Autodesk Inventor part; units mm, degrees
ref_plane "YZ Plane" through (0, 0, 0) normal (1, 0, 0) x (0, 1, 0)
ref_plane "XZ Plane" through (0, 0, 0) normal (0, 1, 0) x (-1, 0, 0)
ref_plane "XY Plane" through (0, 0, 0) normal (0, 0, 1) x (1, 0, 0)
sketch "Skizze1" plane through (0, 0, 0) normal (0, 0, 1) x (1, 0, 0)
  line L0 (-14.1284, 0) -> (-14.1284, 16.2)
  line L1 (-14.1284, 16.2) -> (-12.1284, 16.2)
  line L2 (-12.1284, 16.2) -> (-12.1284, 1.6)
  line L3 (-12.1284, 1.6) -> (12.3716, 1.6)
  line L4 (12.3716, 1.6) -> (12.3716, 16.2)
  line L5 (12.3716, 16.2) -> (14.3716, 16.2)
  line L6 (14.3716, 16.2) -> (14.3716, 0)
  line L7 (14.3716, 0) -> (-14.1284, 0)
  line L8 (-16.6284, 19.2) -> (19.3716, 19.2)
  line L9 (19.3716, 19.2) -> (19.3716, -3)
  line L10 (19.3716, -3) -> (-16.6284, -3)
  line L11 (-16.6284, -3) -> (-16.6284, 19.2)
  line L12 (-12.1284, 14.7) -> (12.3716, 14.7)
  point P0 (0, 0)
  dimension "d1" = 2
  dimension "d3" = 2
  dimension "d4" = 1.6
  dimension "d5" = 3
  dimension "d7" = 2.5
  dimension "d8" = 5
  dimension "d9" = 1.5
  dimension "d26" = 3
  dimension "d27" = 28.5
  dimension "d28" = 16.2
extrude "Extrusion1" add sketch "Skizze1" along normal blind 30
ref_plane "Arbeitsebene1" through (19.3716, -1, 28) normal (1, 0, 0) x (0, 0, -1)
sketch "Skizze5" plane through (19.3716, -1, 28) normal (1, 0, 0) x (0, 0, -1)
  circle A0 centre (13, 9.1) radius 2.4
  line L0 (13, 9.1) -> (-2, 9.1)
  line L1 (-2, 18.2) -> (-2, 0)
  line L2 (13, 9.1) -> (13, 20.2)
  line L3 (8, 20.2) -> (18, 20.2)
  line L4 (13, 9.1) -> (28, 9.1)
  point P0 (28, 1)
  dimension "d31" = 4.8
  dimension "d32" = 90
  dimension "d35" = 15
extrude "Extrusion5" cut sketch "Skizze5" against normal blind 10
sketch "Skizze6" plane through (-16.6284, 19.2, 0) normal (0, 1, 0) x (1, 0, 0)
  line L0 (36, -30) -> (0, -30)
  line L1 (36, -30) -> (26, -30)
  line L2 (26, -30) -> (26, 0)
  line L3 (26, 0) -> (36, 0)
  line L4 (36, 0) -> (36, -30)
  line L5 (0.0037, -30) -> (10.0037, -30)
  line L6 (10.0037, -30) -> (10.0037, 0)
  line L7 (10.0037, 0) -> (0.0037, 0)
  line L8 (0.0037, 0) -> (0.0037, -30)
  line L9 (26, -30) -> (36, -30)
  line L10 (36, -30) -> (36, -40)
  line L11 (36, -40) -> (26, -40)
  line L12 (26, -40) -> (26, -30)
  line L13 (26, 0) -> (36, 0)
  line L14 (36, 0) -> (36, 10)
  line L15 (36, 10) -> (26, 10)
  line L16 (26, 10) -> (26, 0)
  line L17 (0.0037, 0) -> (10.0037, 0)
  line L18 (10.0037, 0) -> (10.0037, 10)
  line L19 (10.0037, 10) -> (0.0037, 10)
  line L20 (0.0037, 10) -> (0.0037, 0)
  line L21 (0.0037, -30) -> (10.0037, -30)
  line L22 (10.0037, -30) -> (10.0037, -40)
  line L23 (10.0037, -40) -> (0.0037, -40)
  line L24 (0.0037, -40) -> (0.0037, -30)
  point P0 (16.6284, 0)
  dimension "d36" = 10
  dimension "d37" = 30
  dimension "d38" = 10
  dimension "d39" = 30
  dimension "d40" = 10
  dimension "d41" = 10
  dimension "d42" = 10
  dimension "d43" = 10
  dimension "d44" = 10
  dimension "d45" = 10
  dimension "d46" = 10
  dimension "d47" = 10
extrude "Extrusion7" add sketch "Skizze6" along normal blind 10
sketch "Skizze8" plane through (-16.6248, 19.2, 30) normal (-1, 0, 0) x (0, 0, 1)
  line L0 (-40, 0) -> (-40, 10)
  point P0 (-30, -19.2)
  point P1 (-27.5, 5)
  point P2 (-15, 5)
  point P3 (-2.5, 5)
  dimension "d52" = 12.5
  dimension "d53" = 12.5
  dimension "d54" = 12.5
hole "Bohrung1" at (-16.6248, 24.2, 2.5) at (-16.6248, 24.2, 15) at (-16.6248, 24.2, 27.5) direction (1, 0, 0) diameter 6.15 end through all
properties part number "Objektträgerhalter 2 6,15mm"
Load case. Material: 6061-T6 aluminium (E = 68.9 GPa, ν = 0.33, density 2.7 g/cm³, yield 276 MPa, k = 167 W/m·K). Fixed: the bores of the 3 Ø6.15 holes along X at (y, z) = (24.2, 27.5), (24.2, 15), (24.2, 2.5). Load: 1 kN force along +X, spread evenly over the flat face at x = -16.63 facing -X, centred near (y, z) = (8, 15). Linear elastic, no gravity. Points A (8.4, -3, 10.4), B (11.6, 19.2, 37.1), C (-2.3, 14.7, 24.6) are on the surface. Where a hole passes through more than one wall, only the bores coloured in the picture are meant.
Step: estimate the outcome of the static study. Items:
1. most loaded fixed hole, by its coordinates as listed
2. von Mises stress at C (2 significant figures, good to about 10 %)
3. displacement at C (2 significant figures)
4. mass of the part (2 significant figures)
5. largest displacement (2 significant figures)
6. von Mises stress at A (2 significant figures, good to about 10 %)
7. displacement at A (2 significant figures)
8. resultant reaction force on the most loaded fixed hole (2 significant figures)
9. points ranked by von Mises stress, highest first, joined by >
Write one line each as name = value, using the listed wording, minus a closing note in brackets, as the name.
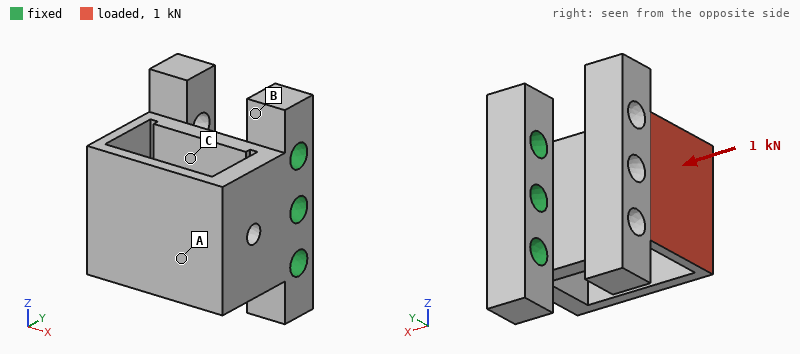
most loaded fixed hole, by its coordinates as listed = (24.2, 15)
von Mises stress at C = 20 MPa
displacement at C = 18 µm
mass of the part = 52 g
largest displacement = 72 µm
von Mises stress at A = 8.5 MPa
displacement at A = 57 µm
resultant reaction force on the most loaded fixed hole = 410 N
points ranked by von Mises stress, highest first, joined by > = C > A > B
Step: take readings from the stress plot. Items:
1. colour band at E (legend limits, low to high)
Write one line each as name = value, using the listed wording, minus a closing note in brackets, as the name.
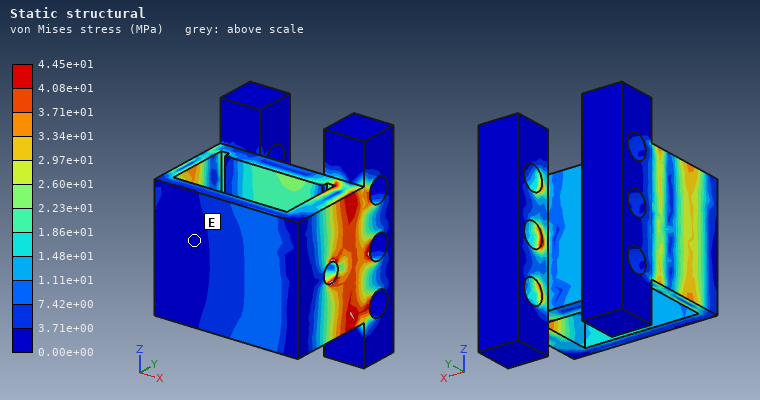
colour band at E = 0.00e+00 to 3.71e+00 MPa
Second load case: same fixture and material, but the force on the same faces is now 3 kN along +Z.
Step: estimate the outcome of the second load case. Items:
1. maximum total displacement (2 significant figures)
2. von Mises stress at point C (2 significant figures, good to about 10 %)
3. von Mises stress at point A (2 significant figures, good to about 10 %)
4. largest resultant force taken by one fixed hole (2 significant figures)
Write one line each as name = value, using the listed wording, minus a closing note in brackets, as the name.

maximum total displacement = 0.27 mm
von Mises stress at point C = 110 MPa
von Mises stress at point A = 41 MPa
largest resultant force taken by one fixed hole = 3.8 kN
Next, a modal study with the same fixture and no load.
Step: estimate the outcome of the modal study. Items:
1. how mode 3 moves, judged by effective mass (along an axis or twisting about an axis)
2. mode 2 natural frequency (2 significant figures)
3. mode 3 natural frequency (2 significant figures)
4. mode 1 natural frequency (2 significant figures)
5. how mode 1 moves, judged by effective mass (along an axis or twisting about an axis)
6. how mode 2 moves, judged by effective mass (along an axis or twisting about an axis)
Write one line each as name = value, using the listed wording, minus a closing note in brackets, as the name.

how mode 3 moves, judged by effective mass = along X
mode 2 natural frequency = 4000 Hz
mode 3 natural frequency = 5900 Hz
mode 1 natural frequency = 2200 Hz
how mode 1 moves, judged by effective mass = along Y
how mode 2 moves, judged by effective mass = twisting about X
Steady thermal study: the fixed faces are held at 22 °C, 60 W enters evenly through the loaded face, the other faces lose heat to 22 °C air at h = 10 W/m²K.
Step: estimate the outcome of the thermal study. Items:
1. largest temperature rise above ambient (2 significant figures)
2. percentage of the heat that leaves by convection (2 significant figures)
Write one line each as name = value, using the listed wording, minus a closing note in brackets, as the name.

largest temperature rise above ambient = 64 K
percentage of the heat that leaves by convection = 4.5 %
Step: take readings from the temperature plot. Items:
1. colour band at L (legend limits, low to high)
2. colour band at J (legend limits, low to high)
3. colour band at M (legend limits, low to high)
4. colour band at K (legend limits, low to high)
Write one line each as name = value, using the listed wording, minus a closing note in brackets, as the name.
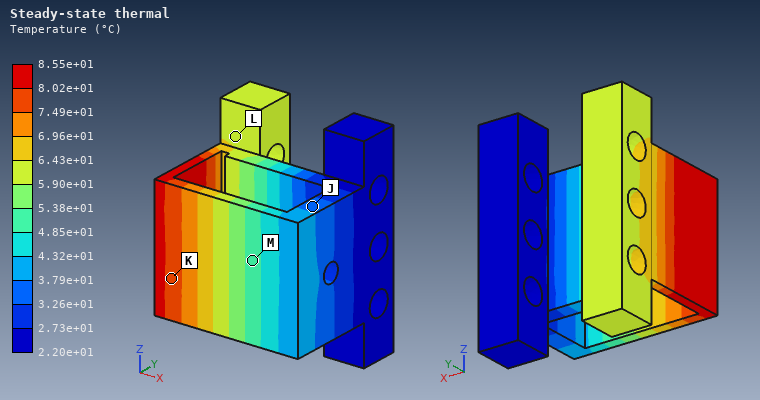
colour band at L = 5.90e+01 to 6.43e+01 °C
colour band at J = 3.26e+01 to 3.79e+01 °C
colour band at M = 4.85e+01 to 5.38e+01 °C
colour band at K = 7.49e+01 to 8.02e+01 °C
